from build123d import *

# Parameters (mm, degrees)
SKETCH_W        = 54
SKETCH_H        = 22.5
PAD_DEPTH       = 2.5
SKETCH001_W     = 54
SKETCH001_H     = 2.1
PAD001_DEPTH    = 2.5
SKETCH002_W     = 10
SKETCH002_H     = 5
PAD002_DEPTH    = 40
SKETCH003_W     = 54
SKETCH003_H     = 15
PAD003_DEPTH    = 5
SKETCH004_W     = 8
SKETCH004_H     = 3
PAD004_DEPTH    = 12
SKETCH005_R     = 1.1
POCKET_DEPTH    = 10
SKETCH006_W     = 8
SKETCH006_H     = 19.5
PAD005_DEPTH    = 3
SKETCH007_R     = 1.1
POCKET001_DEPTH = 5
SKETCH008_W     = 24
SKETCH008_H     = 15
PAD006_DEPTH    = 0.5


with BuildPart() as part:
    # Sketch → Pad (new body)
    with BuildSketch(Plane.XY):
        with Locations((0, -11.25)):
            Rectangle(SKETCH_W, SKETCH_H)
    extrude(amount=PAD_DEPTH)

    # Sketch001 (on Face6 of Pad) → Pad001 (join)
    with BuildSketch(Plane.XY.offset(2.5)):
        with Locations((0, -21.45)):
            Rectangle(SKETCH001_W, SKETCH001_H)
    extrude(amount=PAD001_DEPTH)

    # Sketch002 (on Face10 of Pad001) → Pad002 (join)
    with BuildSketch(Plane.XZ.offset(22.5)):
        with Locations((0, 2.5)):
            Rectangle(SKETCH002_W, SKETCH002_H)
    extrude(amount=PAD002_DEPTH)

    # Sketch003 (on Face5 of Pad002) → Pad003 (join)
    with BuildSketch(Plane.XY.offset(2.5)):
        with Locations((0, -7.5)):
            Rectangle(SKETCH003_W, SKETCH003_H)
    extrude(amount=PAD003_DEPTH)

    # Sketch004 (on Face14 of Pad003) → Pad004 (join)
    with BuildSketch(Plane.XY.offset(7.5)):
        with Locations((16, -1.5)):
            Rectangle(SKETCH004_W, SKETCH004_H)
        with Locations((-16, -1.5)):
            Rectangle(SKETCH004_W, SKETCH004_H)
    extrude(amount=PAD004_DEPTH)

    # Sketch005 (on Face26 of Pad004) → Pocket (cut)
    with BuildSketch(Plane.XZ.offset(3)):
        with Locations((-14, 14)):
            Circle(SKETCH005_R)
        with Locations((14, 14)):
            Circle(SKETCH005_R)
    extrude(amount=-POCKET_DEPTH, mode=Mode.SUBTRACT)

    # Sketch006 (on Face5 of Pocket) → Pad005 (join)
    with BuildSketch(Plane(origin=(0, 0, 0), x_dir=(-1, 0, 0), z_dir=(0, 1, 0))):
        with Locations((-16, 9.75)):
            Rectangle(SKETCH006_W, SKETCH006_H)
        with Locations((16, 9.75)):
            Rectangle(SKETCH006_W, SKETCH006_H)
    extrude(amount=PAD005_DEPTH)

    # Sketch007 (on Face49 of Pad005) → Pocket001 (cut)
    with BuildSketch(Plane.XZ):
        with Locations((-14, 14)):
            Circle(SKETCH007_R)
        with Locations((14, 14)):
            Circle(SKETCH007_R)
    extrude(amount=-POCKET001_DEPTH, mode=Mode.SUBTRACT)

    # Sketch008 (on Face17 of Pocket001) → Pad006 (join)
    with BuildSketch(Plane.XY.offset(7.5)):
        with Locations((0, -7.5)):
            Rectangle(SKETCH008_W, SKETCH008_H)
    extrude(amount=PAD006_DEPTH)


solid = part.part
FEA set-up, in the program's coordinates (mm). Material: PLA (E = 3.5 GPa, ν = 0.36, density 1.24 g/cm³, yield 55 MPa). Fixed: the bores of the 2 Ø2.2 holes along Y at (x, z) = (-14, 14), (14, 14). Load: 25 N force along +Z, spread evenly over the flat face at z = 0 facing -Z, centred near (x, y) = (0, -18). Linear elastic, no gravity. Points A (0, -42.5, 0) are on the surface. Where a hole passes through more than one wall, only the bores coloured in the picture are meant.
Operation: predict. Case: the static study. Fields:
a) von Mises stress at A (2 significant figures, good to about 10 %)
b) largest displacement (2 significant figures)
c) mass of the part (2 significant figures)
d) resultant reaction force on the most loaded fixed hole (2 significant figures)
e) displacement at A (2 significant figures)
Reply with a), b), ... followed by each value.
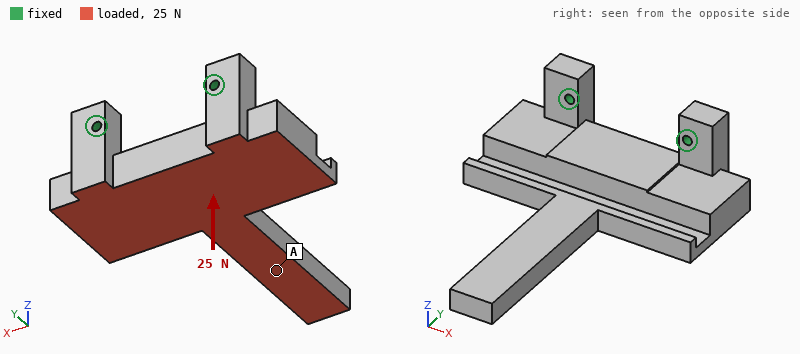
a) 0.74 MPa
b) 0.88 mm
c) 14 g
d) 13 N
e) 0.51 mm
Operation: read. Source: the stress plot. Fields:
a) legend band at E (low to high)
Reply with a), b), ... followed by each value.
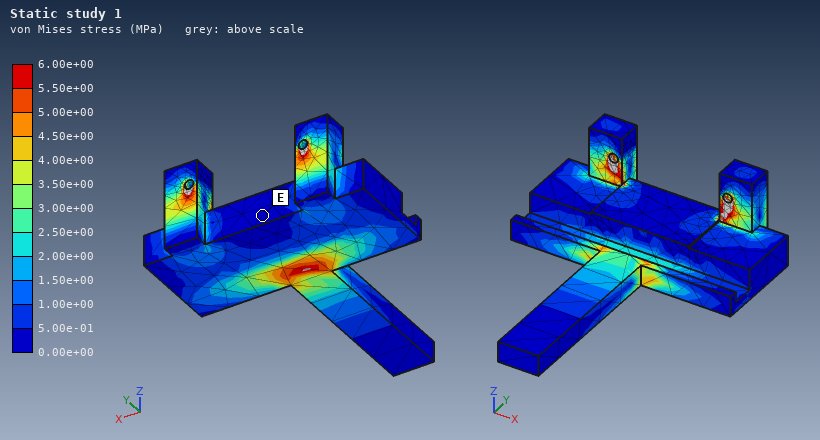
a) 0.00e+00 to 5.00e-01 MPa
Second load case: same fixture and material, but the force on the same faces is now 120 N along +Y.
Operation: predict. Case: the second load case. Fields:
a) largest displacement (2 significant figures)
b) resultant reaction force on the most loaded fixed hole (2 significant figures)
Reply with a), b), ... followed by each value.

a) 1.0 mm
b) 60 N
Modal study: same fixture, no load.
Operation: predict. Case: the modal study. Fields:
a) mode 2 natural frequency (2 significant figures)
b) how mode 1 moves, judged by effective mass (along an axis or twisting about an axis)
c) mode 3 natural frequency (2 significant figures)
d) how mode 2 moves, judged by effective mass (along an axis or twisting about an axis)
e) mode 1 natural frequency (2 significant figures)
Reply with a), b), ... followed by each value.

a) 1100 Hz
b) along Z
c) 1300 Hz
d) along X
e) 350 Hz
